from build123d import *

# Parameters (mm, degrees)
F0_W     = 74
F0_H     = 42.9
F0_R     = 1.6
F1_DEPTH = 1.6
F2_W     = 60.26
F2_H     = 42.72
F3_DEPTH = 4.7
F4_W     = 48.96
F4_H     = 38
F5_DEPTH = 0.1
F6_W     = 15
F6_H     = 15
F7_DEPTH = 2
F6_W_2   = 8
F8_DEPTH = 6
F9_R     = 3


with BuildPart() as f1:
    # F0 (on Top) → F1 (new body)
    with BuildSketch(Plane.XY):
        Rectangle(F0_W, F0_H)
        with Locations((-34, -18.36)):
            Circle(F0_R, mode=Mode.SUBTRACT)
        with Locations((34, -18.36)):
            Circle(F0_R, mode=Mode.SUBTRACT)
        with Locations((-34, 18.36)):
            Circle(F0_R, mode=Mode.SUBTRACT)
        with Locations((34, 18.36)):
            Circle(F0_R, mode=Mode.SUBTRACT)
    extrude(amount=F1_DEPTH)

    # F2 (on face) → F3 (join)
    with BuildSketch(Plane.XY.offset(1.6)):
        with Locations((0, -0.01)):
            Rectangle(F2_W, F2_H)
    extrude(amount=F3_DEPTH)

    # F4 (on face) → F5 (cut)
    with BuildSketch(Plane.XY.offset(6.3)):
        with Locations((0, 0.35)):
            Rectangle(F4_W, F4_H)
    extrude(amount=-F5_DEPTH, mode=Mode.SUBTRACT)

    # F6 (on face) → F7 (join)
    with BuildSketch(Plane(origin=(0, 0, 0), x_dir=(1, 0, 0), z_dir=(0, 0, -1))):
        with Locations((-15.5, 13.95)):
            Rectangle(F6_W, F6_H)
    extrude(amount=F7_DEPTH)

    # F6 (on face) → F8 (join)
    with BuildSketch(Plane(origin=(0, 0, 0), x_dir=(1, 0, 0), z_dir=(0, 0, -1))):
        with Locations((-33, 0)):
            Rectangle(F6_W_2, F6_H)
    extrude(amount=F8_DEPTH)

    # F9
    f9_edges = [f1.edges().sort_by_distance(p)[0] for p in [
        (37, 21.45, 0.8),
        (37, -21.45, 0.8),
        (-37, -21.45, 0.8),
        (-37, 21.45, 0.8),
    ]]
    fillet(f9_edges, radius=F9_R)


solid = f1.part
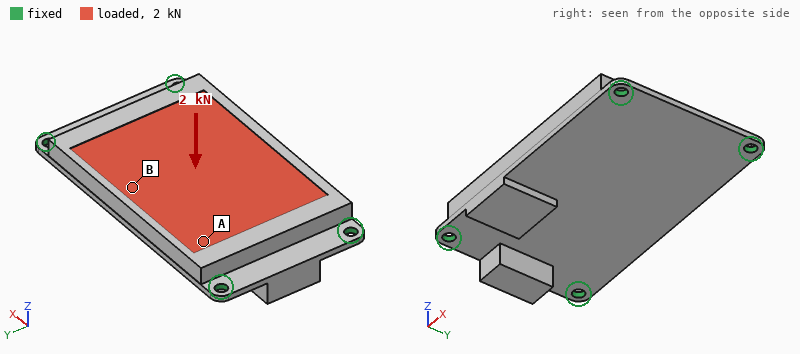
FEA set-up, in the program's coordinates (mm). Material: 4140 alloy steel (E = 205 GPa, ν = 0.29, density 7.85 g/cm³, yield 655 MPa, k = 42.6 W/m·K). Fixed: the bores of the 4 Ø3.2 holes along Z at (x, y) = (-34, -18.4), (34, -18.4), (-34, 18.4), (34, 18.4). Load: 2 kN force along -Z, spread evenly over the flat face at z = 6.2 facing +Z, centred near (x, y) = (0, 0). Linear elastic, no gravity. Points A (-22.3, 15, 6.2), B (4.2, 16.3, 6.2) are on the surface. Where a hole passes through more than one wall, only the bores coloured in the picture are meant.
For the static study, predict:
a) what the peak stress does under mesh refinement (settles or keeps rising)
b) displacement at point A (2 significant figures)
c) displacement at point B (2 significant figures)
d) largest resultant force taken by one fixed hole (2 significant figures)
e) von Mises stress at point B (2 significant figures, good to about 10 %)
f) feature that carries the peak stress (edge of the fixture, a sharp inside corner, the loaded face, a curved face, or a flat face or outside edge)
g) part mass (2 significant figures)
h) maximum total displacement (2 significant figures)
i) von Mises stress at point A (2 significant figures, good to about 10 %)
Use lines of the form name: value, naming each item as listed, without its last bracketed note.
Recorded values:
what the peak stress does under mesh refinement: keeps rising
displacement at point A: 19 µm
displacement at point B: 35 µm
largest resultant force taken by one fixed hole: 1.2 kN
von Mises stress at point B: 57 MPa
feature that carries the peak stress: edge of the fixture
part mass: 140 g
maximum total displacement: 37 µm
von Mises stress at point A: 30 MPa
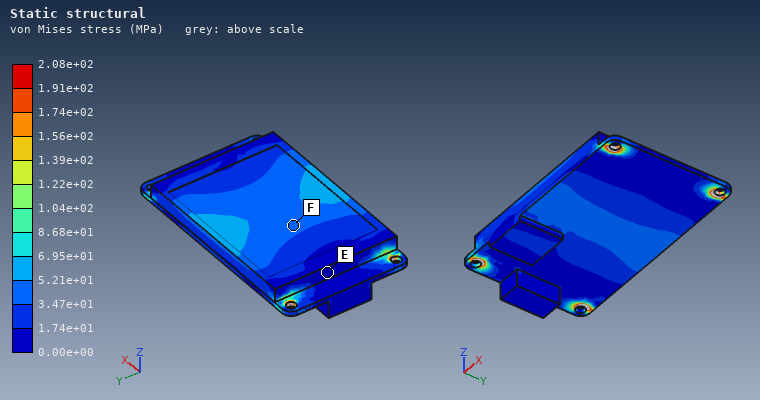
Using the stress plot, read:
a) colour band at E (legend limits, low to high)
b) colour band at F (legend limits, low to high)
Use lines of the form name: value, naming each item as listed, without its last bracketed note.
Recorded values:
colour band at E: 0.00e+00 to 1.74e+01 MPa
colour band at F: 3.47e+01 to 5.21e+01 MPa
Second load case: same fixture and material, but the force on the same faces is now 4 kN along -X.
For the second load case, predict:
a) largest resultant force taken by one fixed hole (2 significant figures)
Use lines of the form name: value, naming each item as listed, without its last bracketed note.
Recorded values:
largest resultant force taken by one fixed hole: 1.1 kN
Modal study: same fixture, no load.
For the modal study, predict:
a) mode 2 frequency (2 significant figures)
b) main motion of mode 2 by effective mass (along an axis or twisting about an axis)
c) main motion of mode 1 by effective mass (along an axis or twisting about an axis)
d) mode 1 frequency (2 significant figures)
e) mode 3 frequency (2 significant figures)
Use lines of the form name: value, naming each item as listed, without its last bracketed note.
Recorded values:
mode 2 frequency: 6800 Hz
main motion of mode 2 by effective mass: twisting about X
main motion of mode 1 by effective mass: along Z
mode 1 frequency: 3900 Hz
mode 3 frequency: 8600 Hz
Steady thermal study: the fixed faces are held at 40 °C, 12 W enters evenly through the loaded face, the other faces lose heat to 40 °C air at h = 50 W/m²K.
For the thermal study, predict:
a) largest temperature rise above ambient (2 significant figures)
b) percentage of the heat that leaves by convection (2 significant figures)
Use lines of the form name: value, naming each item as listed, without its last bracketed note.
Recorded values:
largest temperature rise above ambient: 21 K
percentage of the heat that leaves by convection: 38 %
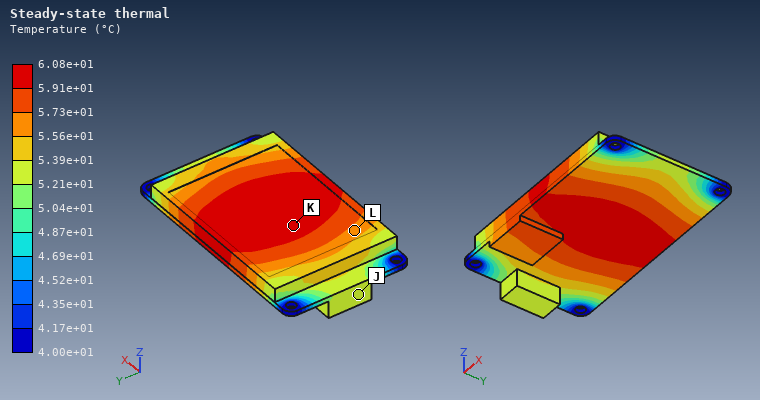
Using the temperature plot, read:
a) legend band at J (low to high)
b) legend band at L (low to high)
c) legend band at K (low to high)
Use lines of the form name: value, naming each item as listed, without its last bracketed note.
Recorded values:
legend band at J: 5.21e+01 to 5.39e+01 °C
legend band at L: 5.56e+01 to 5.73e+01 °C
legend band at K: 5.91e+01 to 6.08e+01 °C
